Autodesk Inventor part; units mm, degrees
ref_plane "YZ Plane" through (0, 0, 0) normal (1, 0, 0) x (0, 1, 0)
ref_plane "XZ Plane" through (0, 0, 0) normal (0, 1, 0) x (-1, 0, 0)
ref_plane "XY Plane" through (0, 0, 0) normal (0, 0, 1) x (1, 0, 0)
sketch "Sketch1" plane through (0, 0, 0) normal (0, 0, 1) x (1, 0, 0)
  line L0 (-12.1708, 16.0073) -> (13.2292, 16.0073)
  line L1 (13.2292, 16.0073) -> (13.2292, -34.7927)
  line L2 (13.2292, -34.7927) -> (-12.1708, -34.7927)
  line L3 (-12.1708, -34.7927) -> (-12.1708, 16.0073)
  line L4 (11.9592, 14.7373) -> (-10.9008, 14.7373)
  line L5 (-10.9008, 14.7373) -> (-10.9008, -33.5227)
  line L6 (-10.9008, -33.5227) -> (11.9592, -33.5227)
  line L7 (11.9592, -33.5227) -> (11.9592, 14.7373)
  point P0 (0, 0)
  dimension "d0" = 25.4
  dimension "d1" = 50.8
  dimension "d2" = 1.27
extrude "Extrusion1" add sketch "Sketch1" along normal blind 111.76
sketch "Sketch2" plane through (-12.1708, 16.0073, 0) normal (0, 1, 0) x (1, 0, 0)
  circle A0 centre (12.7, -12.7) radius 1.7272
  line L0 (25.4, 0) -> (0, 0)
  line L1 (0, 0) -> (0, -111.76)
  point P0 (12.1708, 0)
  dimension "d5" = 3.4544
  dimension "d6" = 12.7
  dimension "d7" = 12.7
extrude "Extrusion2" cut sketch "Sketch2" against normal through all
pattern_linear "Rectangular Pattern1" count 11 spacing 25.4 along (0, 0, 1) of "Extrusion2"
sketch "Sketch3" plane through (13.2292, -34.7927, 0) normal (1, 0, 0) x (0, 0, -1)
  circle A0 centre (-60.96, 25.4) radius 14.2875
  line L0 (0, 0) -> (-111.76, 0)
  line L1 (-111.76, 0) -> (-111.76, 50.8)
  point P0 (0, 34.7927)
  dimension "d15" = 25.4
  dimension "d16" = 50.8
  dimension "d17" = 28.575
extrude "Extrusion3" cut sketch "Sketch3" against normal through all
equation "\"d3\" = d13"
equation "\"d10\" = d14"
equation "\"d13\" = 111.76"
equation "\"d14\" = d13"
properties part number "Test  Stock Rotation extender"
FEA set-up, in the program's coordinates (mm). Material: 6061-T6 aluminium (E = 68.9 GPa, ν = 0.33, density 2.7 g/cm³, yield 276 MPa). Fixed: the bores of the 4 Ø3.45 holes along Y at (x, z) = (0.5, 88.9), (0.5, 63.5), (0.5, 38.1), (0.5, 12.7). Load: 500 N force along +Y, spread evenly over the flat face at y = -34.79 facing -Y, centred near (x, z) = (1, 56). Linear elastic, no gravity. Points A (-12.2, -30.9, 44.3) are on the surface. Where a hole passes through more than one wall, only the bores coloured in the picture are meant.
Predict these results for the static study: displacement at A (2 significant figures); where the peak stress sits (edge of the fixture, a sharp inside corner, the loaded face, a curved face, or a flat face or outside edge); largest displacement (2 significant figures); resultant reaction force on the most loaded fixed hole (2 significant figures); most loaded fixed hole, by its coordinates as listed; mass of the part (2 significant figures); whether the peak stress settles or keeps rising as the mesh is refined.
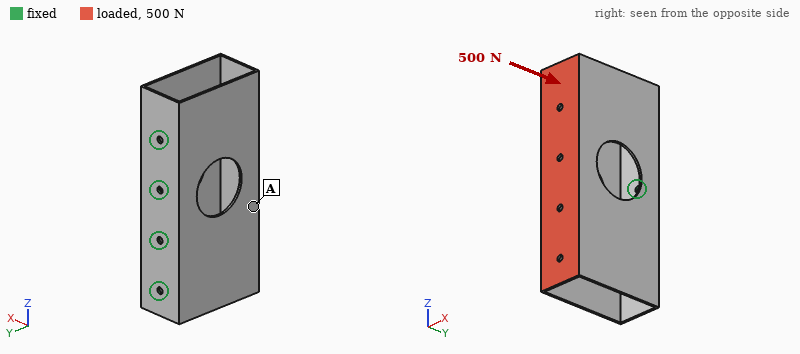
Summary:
0.077 mm
edge of the fixture
0.15 mm
170 N
(0.5, 88.9)
52 g
keeps rising
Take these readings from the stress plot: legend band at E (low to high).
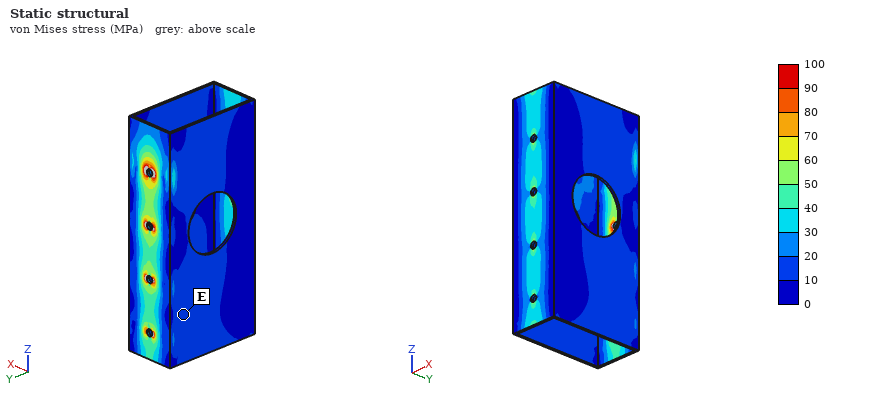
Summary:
10 to 20 MPa
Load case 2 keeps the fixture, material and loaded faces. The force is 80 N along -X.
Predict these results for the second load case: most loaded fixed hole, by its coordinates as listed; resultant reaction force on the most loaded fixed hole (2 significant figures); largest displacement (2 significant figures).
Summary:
(0.5, 88.9)
36 N
1.0 mm
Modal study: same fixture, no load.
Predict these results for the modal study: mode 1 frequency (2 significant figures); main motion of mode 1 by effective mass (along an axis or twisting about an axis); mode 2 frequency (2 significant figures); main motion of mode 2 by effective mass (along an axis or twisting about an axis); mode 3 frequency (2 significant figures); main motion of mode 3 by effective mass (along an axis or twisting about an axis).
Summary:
310 Hz
along X
1000 Hz
twisting about Y
1200 Hz
along Z
